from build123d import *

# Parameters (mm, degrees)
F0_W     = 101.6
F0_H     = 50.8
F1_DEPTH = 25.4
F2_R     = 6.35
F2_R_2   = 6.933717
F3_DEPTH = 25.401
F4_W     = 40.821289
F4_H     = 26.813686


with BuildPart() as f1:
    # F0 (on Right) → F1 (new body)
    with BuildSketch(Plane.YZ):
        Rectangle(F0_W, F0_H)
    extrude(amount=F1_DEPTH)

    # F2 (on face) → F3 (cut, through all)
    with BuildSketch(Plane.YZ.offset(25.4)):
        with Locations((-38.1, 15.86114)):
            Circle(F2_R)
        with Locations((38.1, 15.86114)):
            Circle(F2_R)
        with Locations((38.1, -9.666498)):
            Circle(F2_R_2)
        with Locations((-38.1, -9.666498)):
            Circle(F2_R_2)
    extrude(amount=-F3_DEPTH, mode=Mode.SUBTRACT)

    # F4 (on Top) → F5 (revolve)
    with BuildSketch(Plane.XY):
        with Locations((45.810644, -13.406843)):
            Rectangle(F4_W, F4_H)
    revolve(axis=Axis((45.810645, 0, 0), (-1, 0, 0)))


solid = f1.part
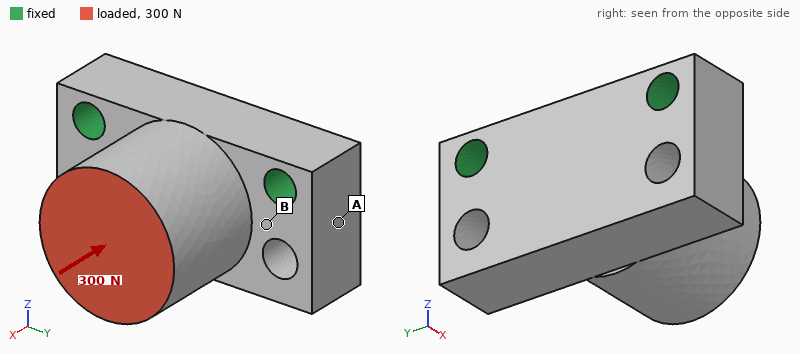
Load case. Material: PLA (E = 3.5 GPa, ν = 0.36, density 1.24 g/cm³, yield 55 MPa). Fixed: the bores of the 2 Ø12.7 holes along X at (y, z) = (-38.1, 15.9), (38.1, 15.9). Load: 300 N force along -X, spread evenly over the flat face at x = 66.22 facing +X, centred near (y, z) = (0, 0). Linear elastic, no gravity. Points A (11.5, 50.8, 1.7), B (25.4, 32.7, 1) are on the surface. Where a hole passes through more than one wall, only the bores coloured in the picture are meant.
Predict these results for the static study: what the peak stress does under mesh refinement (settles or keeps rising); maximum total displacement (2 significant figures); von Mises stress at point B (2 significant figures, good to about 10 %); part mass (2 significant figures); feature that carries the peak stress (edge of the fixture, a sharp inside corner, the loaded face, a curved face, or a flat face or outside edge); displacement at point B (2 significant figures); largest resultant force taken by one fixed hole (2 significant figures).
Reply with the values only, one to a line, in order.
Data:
keeps rising
18 µm
0.50 MPa
260 g
edge of the fixture
3.7 µm
150 N
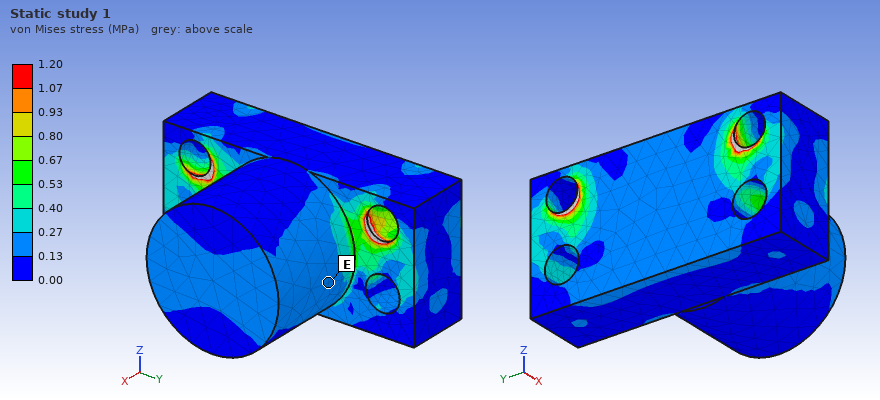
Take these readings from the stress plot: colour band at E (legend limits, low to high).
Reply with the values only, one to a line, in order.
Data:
0.13 to 0.27 MPa
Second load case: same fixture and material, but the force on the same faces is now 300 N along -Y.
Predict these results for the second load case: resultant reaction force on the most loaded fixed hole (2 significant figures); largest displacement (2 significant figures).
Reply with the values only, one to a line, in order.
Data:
280 N
24 µm
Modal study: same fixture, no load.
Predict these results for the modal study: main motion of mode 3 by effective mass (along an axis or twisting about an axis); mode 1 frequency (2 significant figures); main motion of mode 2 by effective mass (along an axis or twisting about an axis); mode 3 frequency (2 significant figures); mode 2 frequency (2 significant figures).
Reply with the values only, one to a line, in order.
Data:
along X
1200 Hz
along Y
3000 Hz
2600 Hz
